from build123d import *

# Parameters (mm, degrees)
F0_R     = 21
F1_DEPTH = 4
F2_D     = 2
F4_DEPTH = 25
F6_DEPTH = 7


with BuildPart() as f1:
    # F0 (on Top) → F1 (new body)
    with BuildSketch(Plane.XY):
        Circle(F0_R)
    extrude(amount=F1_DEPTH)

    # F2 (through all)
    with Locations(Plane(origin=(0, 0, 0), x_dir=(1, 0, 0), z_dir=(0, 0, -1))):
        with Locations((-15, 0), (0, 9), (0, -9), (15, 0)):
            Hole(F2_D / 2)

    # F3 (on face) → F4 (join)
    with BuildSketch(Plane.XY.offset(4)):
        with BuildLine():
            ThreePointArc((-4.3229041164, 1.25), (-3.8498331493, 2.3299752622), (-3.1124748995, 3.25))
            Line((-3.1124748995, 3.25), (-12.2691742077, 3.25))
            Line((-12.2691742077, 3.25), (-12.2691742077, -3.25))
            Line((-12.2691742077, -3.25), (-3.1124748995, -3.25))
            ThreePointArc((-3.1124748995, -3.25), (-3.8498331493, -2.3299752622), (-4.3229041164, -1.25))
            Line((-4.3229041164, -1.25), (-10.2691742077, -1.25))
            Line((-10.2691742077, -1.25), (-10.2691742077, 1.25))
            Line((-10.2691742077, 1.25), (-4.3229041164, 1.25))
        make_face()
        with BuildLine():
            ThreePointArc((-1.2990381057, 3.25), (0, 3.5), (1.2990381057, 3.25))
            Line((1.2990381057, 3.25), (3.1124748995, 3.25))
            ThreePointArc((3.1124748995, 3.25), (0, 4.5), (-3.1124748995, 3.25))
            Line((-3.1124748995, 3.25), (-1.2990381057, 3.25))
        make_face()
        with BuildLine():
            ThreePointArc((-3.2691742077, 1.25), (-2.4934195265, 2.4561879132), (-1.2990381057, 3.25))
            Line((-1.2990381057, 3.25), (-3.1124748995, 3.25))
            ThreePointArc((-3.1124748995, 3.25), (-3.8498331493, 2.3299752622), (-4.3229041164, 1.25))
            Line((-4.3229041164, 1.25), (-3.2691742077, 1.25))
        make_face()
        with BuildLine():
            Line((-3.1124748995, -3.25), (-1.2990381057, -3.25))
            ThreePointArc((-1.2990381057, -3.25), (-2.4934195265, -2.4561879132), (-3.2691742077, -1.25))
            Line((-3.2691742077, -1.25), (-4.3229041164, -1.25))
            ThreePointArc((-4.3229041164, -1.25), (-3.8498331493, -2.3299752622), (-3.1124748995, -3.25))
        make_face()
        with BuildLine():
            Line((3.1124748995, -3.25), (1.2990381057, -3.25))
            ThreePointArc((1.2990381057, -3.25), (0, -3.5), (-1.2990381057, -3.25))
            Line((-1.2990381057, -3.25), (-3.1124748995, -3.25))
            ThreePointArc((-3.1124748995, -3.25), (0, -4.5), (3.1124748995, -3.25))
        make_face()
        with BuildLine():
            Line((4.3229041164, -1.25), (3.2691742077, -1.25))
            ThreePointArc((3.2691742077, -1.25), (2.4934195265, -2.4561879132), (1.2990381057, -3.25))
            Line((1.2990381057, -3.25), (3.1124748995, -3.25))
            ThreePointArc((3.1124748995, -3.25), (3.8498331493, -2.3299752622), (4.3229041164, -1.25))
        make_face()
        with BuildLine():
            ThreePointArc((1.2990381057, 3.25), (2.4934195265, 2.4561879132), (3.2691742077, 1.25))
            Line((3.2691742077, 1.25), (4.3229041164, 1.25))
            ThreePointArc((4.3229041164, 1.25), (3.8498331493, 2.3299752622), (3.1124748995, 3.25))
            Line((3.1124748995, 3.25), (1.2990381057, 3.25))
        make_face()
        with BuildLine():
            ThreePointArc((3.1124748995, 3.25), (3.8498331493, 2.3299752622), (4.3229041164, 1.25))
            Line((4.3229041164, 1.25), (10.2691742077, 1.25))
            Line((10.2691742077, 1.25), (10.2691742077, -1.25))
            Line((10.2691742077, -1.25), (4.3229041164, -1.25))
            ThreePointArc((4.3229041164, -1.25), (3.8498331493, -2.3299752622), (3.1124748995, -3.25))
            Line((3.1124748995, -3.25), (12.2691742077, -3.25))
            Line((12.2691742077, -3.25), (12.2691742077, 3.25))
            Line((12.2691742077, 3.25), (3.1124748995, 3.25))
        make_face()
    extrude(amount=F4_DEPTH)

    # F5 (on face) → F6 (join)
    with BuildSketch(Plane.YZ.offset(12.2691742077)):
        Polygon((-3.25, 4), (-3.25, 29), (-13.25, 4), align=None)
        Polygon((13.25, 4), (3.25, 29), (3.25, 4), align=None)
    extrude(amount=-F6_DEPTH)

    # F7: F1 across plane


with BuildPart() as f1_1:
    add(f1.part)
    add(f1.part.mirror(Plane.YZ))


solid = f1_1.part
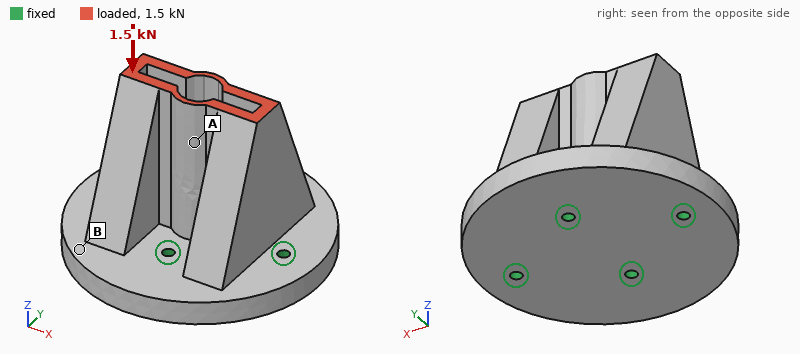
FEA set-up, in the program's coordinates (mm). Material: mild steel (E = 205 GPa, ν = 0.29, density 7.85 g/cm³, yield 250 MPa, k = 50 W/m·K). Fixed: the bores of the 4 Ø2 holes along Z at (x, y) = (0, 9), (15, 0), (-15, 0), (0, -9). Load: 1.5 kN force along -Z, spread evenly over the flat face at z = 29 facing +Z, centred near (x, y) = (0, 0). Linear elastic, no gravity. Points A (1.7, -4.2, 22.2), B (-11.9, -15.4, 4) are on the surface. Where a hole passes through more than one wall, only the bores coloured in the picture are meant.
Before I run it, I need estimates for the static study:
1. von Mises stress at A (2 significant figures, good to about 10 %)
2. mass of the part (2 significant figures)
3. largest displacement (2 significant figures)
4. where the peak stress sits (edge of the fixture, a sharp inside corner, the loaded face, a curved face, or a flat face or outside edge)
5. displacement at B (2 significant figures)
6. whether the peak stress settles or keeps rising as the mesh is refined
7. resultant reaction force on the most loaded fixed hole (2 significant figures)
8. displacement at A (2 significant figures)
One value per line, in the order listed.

12 MPa
90 g
2.3 µm
edge of the fixture
0.96 µm
keeps rising
390 N
1.5 µm
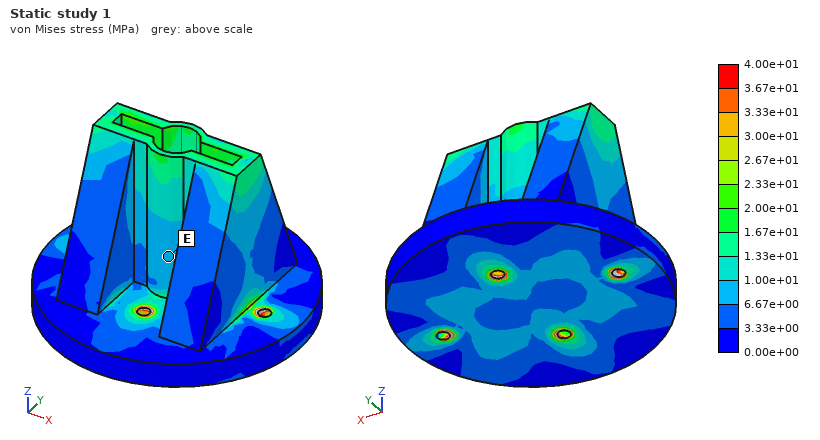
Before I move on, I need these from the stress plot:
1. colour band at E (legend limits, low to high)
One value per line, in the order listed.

6.67e+00 to 1.00e+01 MPa
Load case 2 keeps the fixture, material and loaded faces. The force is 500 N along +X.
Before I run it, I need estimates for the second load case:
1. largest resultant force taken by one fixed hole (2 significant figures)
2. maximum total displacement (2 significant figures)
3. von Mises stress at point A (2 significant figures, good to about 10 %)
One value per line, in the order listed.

480 N
5.5 µm
20 MPa
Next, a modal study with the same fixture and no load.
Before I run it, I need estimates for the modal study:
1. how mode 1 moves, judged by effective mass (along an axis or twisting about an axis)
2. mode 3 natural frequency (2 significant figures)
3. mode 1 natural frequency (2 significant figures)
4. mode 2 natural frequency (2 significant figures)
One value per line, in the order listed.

along Y
14 kHz
11 kHz
14 kHz
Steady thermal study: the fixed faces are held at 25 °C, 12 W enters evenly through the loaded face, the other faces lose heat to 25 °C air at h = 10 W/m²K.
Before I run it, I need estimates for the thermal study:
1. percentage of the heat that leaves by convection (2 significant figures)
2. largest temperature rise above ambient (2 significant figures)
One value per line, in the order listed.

6.0 %
37 K
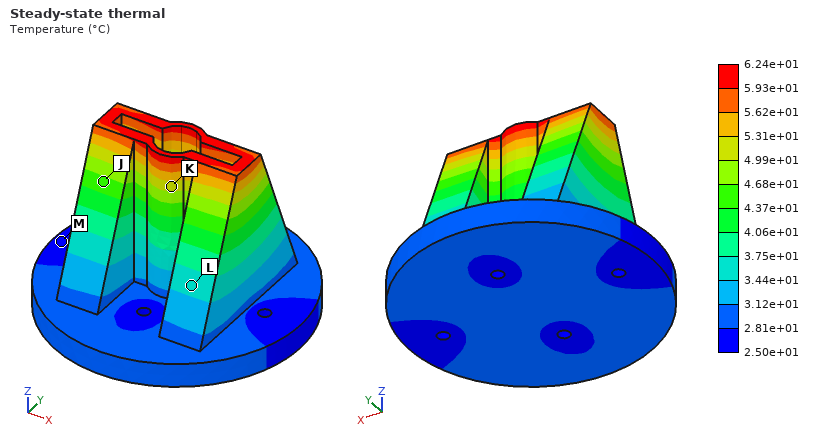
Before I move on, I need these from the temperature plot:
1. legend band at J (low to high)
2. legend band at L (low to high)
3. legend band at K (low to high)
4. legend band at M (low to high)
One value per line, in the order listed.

4.37e+01 to 4.68e+01 °C
3.44e+01 to 3.75e+01 °C
4.99e+01 to 5.31e+01 °C
2.50e+01 to 2.81e+01 °C
